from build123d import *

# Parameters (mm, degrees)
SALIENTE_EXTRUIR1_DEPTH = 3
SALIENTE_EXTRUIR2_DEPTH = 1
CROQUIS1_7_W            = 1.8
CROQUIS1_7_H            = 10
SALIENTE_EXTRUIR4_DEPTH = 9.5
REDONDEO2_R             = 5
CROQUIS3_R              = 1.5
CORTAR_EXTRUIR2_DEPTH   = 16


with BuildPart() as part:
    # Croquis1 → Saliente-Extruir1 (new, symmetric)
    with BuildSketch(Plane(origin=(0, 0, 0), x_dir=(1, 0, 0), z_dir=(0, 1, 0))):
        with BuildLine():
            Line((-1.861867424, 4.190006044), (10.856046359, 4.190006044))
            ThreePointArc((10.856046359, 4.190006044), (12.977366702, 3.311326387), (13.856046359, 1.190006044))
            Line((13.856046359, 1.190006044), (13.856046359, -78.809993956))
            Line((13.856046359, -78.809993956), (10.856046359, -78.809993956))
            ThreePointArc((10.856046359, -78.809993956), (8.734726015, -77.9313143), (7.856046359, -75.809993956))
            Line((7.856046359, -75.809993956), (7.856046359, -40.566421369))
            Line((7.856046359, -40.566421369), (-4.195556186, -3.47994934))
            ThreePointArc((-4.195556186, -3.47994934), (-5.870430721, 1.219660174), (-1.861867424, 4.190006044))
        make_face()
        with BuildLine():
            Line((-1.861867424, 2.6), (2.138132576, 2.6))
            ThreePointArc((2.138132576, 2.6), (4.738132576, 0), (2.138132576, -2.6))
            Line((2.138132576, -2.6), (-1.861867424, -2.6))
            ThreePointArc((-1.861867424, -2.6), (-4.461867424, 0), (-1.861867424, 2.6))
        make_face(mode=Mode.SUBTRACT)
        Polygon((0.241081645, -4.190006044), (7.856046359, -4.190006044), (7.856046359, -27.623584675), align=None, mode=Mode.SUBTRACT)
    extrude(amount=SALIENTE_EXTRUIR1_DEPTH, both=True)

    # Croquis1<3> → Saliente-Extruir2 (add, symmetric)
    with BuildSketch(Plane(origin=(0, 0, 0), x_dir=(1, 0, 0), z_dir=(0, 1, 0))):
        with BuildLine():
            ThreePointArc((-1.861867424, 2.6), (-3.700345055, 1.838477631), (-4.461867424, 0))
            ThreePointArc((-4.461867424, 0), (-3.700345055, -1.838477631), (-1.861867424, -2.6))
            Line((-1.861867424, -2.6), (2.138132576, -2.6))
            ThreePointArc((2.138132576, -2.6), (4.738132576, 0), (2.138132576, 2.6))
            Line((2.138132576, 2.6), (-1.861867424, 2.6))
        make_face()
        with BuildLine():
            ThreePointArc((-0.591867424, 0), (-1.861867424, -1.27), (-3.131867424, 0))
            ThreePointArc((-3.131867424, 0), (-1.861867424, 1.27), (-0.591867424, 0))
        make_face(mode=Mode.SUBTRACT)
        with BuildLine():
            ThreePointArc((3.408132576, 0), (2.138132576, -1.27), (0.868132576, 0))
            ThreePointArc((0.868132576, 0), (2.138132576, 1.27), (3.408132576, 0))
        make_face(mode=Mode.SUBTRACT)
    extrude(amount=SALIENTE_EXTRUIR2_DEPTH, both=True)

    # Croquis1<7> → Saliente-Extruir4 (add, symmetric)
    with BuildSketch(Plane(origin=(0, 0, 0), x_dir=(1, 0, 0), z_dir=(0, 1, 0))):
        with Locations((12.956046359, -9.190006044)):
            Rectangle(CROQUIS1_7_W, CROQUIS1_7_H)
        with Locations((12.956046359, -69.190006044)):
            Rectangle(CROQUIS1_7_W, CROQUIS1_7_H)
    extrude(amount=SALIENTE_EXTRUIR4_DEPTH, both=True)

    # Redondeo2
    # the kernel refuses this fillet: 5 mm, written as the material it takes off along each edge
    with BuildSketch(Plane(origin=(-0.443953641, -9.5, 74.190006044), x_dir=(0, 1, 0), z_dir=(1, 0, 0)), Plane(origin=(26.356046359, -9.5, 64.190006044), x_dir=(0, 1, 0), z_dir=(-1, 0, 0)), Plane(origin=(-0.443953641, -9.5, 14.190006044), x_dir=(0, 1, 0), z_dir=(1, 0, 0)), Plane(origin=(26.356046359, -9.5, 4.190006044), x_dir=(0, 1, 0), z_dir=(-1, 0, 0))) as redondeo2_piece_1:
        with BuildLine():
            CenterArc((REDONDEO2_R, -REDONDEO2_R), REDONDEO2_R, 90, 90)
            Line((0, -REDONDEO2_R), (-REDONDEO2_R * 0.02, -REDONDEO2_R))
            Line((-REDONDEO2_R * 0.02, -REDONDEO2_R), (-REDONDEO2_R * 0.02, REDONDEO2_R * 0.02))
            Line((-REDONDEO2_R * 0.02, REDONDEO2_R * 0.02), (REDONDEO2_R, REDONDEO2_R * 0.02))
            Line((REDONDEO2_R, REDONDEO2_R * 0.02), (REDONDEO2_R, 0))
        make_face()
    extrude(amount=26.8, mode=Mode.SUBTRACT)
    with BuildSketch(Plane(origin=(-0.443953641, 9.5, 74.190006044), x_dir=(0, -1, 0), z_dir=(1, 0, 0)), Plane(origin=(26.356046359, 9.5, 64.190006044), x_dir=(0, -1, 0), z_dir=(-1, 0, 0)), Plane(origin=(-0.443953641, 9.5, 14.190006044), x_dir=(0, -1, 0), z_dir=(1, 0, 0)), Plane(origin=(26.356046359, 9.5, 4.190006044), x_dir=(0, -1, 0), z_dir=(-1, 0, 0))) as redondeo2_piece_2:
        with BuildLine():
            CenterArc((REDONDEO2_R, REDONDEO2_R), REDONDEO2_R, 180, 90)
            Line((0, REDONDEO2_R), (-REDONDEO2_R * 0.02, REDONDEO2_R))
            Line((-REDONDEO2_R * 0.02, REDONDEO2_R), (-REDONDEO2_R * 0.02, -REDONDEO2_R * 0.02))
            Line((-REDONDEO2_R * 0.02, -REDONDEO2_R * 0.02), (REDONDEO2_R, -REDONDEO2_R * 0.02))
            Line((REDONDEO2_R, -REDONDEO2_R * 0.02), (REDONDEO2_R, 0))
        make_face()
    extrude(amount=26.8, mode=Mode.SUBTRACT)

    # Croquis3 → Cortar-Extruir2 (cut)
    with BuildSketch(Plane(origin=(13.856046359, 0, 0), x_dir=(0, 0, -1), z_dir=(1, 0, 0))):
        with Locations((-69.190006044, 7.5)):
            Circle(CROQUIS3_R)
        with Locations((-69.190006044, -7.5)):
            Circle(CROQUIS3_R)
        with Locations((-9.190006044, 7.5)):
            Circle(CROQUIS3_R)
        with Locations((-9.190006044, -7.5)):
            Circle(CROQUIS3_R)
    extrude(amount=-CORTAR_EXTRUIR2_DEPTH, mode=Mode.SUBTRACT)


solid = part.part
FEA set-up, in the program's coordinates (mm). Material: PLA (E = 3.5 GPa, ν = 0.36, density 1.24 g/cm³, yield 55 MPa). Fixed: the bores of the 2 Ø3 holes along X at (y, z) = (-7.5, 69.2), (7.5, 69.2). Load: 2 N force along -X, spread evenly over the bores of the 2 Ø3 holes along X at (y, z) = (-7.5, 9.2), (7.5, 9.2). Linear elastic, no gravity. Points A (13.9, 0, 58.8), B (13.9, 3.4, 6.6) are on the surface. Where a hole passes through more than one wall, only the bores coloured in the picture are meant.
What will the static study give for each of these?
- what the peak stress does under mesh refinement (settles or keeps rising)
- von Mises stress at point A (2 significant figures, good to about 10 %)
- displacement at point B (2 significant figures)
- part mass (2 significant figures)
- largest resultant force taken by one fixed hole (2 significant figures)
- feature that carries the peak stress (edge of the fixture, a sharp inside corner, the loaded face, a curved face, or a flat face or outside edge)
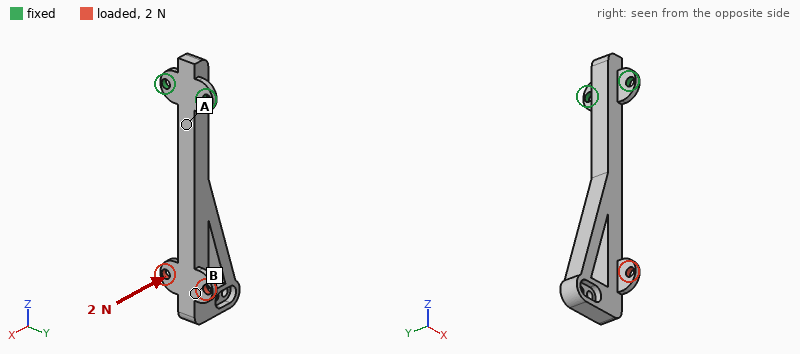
keeps rising
2.8 MPa
0.82 mm
5.6 g
4.1 N
edge of the fixture
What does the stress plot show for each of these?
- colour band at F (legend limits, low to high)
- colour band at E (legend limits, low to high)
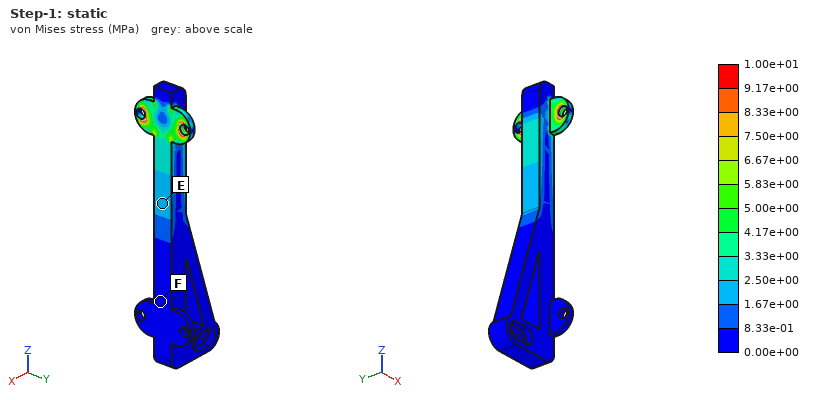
0.00e+00 to 8.33e-01 MPa
1.67e+00 to 2.50e+00 MPa
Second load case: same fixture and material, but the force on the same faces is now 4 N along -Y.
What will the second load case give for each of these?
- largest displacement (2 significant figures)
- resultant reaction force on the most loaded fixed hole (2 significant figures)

0.94 mm
17 N
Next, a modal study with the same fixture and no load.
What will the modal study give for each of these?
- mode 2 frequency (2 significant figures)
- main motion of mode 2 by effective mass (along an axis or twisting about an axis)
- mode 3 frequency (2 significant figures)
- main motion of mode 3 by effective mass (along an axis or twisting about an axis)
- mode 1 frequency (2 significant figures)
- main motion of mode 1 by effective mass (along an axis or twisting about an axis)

210 Hz
along Y
1100 Hz
twisting about Z
140 Hz
along X
